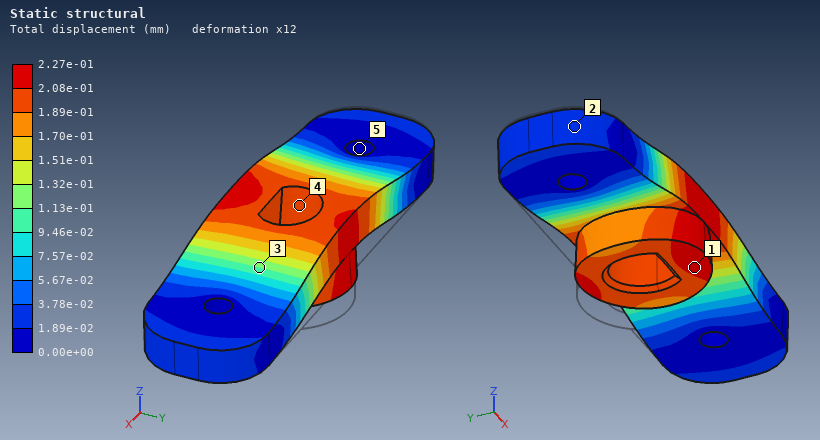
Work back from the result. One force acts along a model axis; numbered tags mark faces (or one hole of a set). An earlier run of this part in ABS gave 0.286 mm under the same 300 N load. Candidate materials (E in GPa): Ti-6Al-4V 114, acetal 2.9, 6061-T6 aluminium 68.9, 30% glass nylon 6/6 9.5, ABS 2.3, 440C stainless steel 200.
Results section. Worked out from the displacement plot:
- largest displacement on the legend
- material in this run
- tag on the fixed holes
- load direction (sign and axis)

2.27e-01 mm
acetal
5
+Z
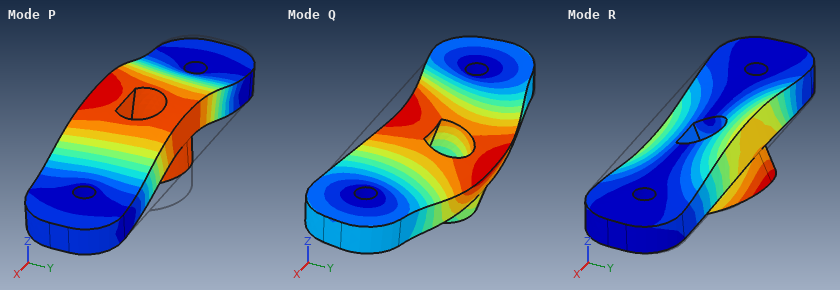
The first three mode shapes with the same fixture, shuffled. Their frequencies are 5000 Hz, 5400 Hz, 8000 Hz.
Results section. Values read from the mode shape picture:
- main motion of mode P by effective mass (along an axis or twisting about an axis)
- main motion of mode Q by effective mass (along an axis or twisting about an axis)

along Z
along Y
